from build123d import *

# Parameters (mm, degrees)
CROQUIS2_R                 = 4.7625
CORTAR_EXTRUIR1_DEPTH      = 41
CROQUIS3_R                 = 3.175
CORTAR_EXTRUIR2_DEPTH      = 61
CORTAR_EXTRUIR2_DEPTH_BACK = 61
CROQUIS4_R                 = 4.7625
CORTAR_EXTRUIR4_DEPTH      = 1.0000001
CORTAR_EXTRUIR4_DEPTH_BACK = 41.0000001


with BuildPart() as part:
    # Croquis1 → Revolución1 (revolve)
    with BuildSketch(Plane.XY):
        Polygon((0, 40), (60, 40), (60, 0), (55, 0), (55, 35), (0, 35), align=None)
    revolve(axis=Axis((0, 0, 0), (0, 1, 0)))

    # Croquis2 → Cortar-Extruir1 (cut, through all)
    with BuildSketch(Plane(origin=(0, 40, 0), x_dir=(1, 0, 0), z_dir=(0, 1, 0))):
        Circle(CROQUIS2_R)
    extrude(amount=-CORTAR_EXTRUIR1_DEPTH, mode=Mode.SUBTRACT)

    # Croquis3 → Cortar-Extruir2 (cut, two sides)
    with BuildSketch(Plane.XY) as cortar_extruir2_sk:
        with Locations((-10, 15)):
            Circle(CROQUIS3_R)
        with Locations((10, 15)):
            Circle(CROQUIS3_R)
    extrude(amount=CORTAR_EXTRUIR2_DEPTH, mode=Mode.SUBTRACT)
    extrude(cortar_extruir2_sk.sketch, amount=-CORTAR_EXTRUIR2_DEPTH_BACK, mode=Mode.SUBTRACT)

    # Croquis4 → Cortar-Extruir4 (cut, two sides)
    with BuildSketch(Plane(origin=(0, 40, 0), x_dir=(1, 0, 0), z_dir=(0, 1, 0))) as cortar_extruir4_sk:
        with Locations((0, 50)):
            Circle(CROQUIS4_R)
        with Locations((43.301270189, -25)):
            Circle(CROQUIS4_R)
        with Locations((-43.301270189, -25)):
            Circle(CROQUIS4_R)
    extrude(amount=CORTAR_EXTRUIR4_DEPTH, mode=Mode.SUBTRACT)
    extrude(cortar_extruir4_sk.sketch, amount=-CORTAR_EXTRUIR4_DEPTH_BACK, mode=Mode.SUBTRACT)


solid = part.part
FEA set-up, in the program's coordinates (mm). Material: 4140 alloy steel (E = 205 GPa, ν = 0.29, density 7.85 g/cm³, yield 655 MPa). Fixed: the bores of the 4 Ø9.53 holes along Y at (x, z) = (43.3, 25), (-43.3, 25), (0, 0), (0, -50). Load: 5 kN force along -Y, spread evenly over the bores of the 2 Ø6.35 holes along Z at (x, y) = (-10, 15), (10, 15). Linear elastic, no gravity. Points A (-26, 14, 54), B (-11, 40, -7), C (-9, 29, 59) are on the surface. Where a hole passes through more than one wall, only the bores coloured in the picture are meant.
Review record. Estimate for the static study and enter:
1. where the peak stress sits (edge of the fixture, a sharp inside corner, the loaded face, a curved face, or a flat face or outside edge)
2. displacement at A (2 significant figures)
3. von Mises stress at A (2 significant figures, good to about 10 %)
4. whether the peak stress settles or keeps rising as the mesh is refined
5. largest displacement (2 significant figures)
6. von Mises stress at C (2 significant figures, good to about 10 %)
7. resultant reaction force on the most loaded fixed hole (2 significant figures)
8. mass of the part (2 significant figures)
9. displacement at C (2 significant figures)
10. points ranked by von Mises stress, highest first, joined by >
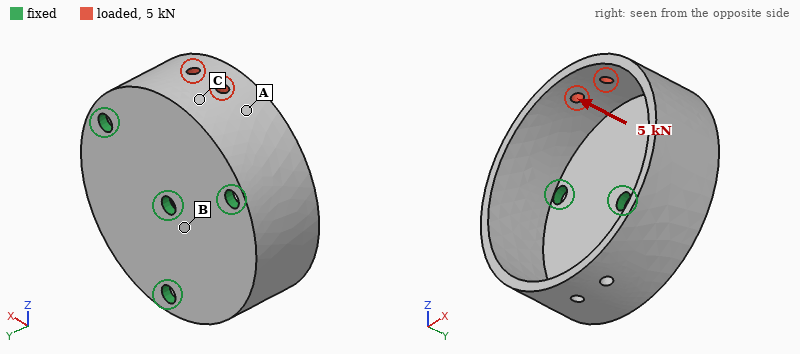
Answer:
edge of the fixture
0.085 mm
78 MPa
keeps rising
0.16 mm
45 MPa
3.0 kN
920 g
0.093 mm
A > C > B
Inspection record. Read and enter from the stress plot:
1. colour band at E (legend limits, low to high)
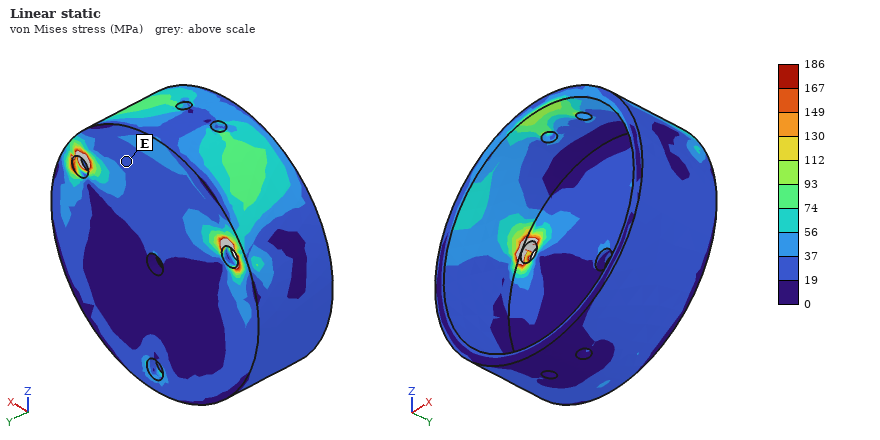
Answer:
19 to 37 MPa
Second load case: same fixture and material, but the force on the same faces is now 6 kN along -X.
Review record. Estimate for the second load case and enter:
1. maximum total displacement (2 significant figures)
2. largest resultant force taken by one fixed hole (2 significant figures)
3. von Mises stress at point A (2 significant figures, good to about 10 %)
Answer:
51 µm
3.8 kN
24 MPa
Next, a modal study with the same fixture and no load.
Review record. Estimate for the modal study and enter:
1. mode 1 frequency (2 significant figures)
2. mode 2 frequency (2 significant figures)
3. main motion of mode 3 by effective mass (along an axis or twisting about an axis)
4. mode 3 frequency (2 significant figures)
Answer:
2300 Hz
2300 Hz
along Y
4100 Hz
